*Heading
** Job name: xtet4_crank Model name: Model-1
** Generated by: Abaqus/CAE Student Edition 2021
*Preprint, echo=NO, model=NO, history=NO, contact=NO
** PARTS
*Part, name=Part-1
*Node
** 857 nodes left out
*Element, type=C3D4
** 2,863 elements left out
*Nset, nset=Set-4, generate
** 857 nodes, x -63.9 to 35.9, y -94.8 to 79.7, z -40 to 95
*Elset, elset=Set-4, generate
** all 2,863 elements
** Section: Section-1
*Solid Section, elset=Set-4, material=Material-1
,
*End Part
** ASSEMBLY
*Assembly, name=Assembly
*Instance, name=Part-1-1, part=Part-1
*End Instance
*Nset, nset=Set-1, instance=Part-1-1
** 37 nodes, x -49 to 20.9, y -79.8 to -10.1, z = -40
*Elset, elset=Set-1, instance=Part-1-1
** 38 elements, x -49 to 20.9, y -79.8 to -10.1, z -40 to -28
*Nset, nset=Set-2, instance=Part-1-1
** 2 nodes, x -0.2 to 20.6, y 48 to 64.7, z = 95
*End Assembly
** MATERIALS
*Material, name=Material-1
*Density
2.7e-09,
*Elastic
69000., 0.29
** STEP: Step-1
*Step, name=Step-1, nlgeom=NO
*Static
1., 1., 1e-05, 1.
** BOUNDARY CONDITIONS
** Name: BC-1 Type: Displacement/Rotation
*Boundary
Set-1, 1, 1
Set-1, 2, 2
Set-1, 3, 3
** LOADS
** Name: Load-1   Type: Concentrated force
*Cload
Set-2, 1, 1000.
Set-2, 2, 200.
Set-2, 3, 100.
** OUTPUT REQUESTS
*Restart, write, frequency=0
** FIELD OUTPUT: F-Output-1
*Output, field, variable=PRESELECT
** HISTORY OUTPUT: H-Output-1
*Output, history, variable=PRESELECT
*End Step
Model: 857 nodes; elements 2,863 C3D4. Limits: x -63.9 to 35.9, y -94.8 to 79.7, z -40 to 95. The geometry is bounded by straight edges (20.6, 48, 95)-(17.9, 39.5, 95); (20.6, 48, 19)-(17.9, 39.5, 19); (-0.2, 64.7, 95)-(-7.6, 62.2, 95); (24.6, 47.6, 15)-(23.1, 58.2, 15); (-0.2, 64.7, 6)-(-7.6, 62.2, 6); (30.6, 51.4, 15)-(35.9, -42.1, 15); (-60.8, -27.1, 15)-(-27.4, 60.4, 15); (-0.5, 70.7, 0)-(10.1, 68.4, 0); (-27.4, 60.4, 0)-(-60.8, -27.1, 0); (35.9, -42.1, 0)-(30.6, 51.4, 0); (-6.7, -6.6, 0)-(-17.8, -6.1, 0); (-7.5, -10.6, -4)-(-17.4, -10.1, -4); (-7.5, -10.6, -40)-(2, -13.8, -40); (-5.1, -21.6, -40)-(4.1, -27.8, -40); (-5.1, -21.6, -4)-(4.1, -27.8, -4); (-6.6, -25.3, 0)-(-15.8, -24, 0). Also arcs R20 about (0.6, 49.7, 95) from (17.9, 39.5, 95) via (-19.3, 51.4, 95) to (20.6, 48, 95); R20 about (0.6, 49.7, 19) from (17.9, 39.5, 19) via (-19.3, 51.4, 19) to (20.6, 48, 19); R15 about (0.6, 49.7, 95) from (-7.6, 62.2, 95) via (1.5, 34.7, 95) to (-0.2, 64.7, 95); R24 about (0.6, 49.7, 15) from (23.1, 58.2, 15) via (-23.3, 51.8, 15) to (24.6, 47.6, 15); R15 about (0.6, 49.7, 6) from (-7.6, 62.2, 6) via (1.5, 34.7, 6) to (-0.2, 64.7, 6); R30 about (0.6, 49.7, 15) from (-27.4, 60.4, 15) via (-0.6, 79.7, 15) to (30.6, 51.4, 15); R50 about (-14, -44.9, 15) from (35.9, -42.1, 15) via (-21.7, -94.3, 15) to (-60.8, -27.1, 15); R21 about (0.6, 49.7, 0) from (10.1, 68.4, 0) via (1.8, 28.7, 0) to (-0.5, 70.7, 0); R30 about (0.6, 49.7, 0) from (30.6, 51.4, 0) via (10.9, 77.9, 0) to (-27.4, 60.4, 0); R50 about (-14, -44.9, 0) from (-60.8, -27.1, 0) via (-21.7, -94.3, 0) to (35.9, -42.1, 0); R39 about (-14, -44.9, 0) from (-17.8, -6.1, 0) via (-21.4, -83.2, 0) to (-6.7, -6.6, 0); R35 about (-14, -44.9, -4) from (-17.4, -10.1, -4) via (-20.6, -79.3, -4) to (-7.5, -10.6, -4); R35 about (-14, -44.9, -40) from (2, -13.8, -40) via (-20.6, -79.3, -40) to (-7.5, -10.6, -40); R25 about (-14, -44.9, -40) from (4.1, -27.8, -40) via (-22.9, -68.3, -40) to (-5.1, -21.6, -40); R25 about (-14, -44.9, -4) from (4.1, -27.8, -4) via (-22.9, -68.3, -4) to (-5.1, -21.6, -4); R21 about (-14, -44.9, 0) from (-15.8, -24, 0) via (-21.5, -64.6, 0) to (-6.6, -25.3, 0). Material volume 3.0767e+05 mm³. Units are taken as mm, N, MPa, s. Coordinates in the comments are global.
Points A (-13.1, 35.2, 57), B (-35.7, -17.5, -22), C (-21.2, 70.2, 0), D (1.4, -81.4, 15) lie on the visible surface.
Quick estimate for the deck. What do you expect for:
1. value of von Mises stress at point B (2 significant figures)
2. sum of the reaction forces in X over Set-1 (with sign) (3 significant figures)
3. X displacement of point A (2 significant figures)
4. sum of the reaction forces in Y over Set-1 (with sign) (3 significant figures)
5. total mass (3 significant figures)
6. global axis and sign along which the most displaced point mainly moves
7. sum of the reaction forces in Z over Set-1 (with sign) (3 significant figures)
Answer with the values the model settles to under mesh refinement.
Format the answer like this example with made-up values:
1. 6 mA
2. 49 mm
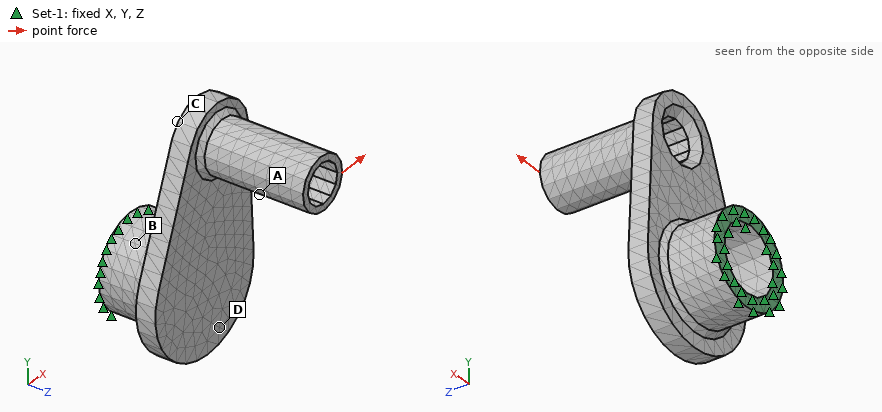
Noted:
1. 14 MPa
2. -2000 N
3. 0.31 mm
4. -400 N
5. 0.831 kg
6. +X
7. -200 N
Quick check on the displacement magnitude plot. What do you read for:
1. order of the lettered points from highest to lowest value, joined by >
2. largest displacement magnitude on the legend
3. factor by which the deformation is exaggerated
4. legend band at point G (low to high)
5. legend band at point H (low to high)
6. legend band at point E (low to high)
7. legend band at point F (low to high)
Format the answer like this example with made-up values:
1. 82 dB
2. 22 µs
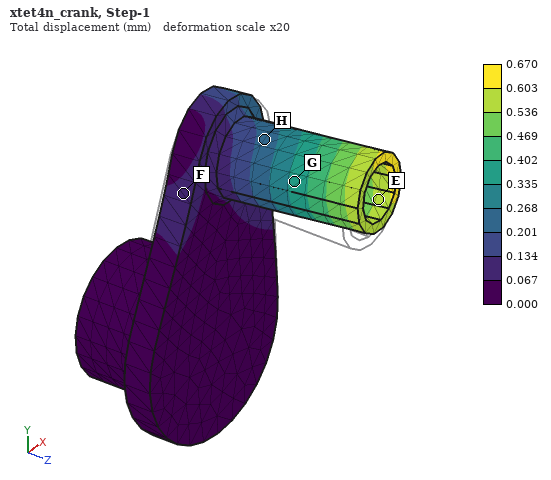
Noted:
1. E > G > H > F
2. 0.670 mm
3. 20
4. 0.335 to 0.402 mm
5. 0.201 to 0.268 mm
6. 0.536 to 0.603 mm
7. 0.067 to 0.134 mm
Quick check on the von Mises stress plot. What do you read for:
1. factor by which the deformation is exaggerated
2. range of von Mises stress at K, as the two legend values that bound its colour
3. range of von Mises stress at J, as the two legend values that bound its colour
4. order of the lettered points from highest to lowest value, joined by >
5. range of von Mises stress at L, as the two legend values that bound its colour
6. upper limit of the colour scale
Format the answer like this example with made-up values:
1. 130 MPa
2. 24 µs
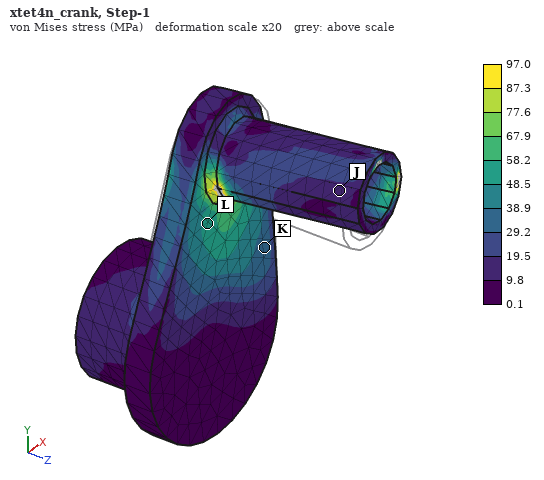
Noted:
1. 20
2. 29.2 to 38.9 MPa
3. 9.8 to 19.5 MPa
4. L > K > J
5. 48.5 to 58.2 MPa
6. 97.0 MPa
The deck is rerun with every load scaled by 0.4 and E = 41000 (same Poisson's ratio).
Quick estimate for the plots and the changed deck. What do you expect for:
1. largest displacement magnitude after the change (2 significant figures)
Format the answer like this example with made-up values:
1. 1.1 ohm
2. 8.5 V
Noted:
1. 0.45 mm
